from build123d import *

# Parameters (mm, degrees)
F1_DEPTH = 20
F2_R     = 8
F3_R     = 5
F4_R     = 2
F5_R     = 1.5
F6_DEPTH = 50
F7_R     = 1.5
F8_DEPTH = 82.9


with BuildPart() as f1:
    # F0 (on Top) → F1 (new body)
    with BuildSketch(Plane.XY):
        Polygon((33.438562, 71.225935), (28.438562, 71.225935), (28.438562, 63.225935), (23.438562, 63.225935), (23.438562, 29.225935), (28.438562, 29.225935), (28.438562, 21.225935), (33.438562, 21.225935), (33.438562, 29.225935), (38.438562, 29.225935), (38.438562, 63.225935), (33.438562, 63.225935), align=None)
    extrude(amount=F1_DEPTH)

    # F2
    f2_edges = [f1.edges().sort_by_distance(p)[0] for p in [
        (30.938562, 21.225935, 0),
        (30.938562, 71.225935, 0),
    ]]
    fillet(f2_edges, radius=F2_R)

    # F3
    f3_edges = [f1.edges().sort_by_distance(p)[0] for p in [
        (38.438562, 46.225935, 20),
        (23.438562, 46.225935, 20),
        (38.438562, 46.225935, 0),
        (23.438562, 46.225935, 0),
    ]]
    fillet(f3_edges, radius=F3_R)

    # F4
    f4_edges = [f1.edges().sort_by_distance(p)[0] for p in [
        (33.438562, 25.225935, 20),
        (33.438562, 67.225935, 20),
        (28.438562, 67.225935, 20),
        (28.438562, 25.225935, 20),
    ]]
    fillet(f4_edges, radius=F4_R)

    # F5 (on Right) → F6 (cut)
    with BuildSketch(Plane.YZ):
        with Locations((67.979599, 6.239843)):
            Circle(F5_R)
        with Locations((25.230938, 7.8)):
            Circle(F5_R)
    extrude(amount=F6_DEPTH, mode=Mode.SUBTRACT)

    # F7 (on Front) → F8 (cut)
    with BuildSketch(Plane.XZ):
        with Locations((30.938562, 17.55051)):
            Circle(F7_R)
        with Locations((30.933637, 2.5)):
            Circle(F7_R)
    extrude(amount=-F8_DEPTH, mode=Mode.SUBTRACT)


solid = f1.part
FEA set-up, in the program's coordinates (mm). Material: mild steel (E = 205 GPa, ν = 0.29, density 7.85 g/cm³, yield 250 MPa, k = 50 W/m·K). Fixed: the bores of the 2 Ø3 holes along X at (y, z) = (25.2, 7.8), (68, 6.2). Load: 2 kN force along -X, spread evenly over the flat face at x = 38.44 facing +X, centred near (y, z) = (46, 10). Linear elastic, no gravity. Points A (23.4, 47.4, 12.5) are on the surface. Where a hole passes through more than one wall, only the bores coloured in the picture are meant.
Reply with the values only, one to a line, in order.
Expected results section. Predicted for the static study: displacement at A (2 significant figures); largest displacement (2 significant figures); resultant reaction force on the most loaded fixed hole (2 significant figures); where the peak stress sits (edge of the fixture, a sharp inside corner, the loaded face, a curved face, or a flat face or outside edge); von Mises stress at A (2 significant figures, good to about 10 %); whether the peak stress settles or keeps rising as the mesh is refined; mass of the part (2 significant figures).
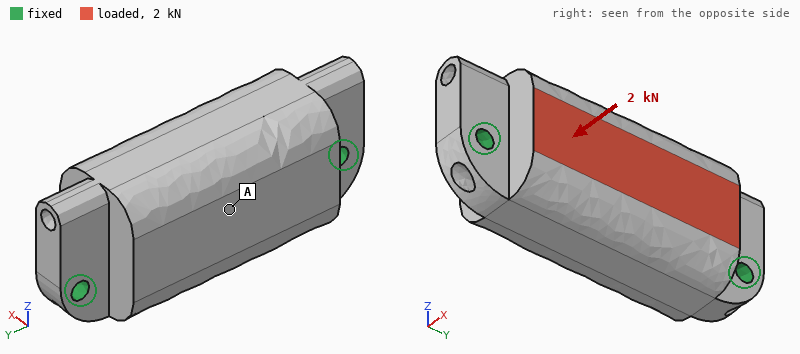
6.0 µm
8.4 µm
1.0 kN
edge of the fixture
16 MPa
keeps rising
80 g
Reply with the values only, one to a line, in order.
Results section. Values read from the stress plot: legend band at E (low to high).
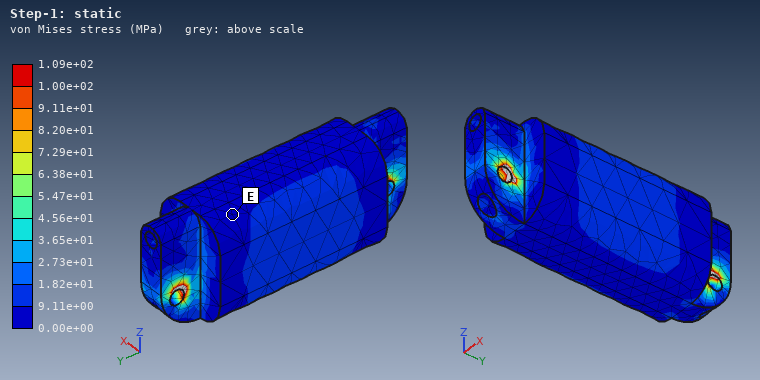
0.00e+00 to 9.11e+00 MPa
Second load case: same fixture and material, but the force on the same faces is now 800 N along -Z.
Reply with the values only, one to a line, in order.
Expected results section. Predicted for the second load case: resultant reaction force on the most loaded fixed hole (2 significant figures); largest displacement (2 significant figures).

420 N
6.6 µm
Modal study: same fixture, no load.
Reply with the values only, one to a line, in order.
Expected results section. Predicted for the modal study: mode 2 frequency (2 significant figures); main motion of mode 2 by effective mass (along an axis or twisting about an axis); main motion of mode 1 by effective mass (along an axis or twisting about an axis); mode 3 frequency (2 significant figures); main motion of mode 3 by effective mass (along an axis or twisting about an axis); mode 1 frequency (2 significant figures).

16 kHz
along X
along X
17 kHz
along Z
8900 Hz
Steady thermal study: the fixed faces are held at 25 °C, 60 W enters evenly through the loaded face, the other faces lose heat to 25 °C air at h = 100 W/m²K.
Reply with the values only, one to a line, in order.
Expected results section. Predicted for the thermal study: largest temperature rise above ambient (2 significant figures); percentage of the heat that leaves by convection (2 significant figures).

73 K
27 %
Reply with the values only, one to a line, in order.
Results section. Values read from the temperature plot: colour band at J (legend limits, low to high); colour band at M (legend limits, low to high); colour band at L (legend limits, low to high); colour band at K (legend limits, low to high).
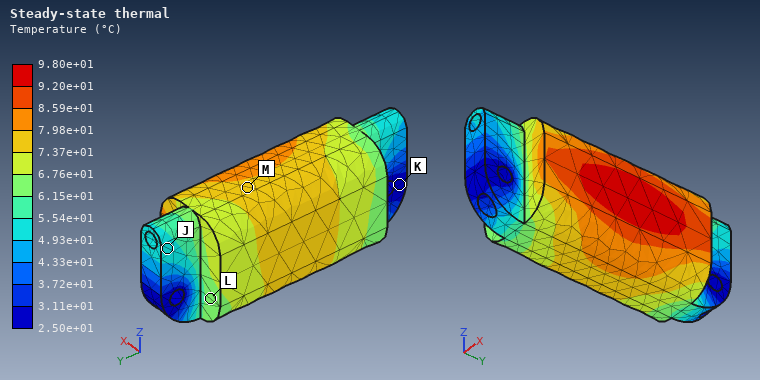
4.93e+01 to 5.54e+01 °C
7.37e+01 to 7.98e+01 °C
6.15e+01 to 6.76e+01 °C
2.50e+01 to 3.11e+01 °C
